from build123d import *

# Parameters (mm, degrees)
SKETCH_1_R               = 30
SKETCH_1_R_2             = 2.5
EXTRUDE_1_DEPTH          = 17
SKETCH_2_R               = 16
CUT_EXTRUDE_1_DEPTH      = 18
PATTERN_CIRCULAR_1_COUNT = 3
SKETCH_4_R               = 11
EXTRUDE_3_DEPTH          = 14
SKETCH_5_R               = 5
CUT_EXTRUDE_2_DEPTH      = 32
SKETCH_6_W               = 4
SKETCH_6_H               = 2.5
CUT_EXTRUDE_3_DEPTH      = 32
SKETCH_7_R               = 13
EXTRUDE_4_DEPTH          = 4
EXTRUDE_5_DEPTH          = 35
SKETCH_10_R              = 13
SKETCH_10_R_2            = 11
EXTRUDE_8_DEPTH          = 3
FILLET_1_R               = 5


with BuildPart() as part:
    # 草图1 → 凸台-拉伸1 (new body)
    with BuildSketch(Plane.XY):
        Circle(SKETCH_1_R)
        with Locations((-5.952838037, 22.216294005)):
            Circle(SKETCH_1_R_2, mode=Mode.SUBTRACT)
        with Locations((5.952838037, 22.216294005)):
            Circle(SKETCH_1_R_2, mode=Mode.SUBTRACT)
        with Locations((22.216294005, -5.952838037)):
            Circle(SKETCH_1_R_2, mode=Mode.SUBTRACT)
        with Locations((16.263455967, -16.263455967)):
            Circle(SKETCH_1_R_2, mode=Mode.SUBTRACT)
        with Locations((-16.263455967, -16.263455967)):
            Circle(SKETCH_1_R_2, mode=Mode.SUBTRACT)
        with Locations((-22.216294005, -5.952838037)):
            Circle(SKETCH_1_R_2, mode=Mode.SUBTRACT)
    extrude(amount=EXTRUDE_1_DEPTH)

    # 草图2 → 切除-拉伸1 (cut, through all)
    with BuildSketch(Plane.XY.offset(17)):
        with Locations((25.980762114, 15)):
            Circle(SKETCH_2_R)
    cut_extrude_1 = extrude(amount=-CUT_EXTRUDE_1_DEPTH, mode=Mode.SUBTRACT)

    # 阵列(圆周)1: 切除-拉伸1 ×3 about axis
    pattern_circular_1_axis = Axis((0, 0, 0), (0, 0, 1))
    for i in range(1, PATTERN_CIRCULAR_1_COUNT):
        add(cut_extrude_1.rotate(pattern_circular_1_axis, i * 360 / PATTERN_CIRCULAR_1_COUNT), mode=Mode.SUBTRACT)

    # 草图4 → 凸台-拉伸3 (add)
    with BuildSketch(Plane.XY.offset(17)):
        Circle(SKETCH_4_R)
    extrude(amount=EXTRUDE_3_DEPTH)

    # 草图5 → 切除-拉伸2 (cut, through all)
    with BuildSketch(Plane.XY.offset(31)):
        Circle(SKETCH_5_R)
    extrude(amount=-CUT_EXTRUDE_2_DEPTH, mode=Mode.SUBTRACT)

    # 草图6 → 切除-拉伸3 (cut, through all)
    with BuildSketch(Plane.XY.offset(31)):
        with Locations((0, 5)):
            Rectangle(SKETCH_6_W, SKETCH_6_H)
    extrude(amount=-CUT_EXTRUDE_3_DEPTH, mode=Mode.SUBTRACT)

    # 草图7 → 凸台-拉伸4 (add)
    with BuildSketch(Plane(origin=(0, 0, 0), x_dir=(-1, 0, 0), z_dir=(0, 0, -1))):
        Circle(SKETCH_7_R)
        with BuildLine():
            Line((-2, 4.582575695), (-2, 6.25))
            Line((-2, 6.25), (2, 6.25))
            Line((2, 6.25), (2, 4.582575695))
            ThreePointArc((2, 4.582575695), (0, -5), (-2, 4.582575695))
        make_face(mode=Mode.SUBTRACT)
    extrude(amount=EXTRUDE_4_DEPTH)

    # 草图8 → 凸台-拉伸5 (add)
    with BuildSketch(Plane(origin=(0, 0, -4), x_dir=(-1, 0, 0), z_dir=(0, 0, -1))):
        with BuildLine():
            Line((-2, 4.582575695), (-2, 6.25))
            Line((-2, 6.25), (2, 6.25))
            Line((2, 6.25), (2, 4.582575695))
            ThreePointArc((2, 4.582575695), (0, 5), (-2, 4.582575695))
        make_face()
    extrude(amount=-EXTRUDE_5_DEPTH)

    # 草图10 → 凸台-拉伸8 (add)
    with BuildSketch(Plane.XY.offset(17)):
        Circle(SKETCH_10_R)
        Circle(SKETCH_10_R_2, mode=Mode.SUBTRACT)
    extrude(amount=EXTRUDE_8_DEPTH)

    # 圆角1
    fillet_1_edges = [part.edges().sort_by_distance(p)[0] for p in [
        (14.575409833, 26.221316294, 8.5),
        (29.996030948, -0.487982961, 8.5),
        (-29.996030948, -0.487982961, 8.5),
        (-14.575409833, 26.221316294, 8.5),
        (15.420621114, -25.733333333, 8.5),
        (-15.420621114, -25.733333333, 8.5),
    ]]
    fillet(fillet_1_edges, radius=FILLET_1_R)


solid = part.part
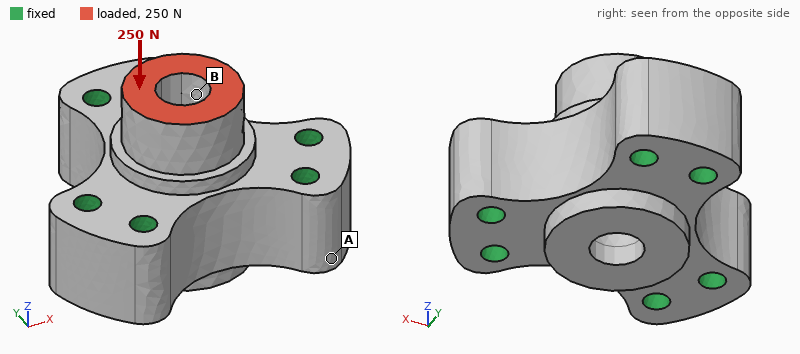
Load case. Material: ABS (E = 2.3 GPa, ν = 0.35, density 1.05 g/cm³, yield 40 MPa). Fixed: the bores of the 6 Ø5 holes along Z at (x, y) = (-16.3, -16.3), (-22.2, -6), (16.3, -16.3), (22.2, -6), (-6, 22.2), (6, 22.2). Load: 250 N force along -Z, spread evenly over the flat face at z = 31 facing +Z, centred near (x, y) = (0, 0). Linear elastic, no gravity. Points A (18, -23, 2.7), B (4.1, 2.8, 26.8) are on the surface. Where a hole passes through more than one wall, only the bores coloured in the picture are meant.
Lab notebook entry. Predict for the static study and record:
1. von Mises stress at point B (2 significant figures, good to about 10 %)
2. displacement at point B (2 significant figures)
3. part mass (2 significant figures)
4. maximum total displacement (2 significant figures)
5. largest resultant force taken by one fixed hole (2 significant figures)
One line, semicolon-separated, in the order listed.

0.76 MPa; 7.8 µm; 34 g; 9.9 µm; 44 N
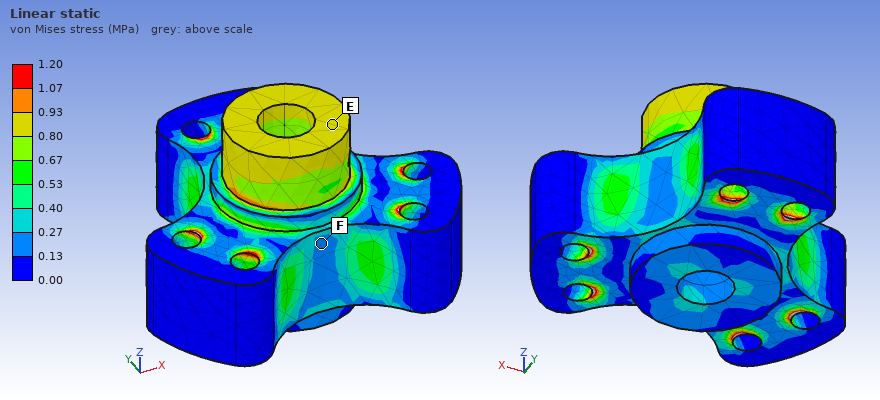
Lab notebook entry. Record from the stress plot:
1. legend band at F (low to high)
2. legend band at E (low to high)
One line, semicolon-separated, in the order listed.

0.13 to 0.27 MPa; 0.80 to 0.93 MPa
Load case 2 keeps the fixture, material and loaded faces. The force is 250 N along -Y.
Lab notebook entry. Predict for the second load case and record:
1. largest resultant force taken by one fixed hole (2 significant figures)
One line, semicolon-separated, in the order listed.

100 N
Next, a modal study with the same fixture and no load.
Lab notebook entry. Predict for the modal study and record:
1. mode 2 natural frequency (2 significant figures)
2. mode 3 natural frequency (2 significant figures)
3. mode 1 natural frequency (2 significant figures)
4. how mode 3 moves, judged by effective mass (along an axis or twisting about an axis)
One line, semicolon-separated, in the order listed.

8400 Hz; 9100 Hz; 8400 Hz; along Z
